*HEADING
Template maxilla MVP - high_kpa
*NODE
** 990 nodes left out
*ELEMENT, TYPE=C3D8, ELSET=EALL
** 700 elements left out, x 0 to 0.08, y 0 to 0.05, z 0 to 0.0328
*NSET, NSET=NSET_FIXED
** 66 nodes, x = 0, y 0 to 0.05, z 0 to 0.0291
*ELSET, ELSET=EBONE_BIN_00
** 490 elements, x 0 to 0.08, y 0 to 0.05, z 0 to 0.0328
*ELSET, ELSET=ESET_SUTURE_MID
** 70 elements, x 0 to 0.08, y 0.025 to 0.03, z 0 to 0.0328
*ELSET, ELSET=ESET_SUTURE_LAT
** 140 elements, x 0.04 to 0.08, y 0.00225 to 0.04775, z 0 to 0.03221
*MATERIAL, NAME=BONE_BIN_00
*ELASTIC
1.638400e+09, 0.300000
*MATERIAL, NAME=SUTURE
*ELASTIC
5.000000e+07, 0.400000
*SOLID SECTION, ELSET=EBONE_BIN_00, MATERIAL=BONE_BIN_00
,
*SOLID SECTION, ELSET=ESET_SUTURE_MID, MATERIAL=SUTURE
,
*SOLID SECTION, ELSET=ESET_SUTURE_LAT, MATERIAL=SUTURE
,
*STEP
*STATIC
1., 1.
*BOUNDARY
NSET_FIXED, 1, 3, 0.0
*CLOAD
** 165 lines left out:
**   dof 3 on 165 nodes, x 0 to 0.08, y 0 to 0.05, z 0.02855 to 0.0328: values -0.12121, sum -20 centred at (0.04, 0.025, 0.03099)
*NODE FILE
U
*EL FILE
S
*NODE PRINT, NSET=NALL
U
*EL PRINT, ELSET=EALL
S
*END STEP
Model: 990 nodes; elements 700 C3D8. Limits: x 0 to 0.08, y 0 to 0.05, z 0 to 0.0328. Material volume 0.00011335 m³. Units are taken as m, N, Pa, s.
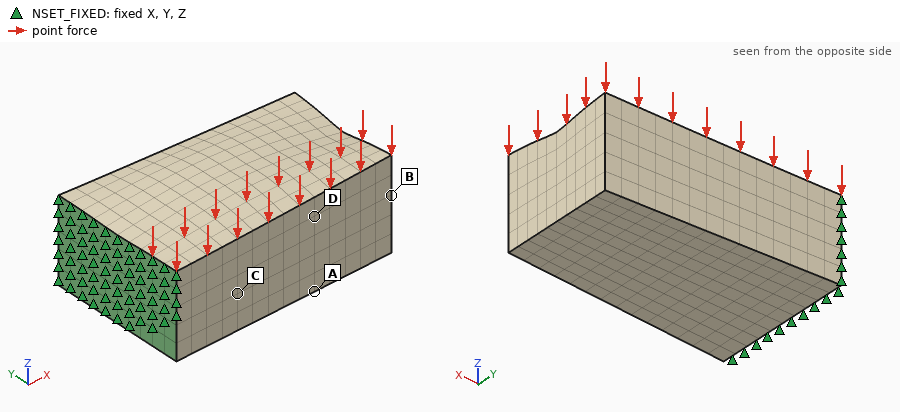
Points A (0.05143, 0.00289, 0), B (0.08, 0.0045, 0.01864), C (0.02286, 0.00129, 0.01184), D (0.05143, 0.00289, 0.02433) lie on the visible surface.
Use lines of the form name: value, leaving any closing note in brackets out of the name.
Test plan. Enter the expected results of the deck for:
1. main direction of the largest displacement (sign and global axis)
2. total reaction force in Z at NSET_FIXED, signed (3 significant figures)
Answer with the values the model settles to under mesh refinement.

main direction of the largest displacement: -Z
total reaction force in Z at NSET_FIXED, signed: 20.0 N
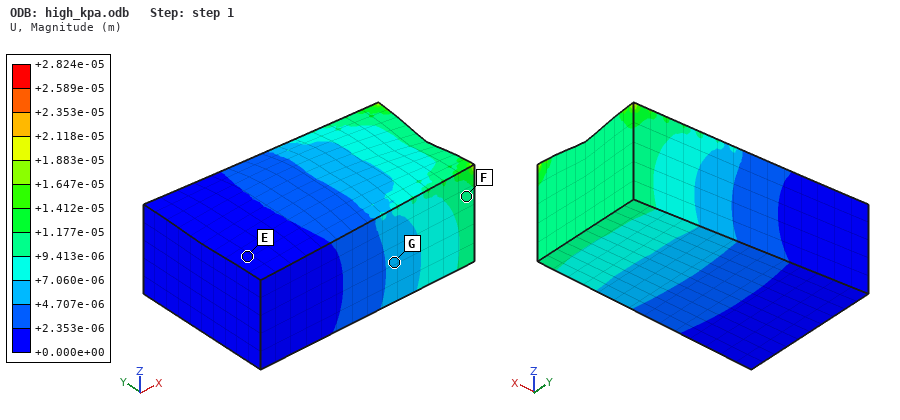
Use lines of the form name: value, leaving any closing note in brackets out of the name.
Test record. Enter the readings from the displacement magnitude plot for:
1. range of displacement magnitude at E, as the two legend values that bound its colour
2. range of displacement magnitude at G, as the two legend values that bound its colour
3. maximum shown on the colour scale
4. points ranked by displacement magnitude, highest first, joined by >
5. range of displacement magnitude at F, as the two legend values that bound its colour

range of displacement magnitude at E, as the two legend values that bound its colour: +0.000e+00 to +2.353e-06 m
range of displacement magnitude at G, as the two legend values that bound its colour: +4.707e-06 to +7.060e-06 m
maximum shown on the colour scale: +2.824e-05 m
points ranked by displacement magnitude, highest first, joined by >: F > G > E
range of displacement magnitude at F, as the two legend values that bound its colour: +9.413e-06 to +1.177e-05 m
